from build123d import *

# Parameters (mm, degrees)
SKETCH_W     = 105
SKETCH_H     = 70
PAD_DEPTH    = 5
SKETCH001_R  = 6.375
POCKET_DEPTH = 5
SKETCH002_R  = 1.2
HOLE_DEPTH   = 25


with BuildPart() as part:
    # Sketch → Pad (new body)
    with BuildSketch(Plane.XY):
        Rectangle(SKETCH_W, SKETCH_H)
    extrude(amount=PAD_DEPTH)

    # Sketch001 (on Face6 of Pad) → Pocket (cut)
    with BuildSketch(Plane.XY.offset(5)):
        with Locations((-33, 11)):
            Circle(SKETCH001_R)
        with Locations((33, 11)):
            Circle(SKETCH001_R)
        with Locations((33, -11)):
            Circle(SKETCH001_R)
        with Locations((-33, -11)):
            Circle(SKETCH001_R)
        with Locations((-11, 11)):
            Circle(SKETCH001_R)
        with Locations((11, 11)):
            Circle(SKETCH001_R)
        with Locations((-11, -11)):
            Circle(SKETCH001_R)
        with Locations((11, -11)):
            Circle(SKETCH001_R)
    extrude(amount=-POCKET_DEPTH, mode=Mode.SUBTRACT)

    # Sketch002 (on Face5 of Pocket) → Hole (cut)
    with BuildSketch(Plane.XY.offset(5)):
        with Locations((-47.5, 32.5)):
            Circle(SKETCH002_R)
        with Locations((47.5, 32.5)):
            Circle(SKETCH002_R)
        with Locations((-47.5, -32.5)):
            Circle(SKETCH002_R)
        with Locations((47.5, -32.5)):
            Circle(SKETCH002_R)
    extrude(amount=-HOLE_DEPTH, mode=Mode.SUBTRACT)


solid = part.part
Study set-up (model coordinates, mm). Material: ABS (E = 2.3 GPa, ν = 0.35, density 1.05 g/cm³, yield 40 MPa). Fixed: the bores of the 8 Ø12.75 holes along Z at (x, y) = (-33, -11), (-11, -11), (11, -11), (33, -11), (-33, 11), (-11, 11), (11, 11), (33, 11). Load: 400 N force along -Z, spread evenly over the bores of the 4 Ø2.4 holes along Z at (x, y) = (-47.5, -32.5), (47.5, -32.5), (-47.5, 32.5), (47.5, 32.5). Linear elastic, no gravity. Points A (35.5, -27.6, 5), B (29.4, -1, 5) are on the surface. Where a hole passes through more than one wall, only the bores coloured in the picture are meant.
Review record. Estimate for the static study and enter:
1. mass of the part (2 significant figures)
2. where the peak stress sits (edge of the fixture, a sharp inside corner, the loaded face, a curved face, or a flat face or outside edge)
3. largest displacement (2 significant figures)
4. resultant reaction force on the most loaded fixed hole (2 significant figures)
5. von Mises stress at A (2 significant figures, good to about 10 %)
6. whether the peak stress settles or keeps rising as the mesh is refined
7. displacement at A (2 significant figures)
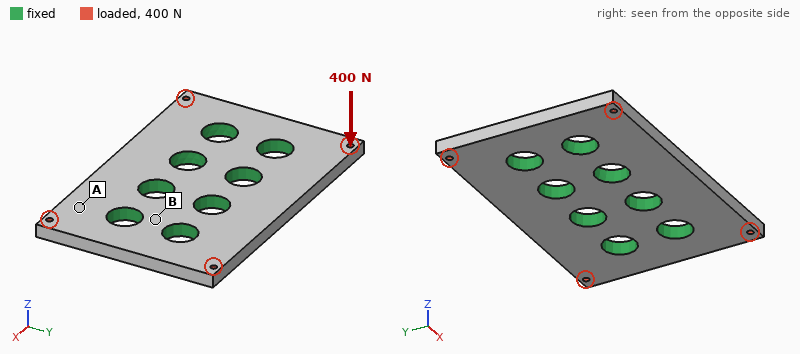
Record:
33 g
edge of the fixture
0.65 mm
120 N
9.1 MPa
keeps rising
0.14 mm
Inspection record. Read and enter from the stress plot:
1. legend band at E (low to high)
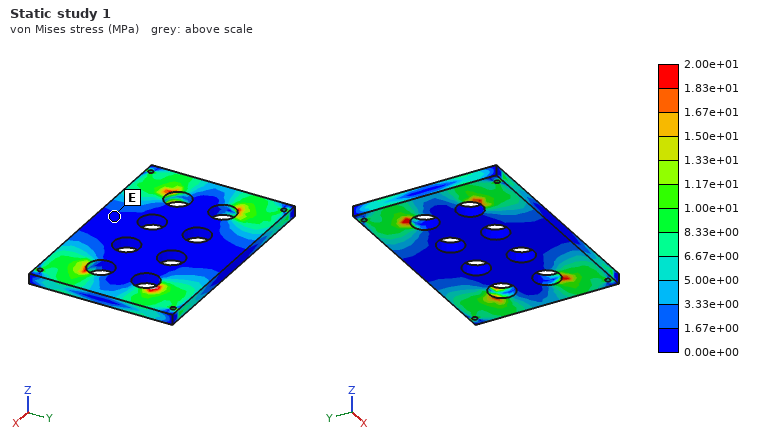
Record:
0.00e+00 to 1.67e+00 MPa
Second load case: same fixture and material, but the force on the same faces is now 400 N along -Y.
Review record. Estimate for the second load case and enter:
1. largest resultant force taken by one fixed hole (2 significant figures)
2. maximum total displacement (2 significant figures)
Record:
110 N
30 µm
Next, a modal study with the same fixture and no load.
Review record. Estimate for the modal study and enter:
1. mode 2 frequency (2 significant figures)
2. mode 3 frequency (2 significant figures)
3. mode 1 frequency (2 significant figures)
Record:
2900 Hz
2900 Hz
2900 Hz
